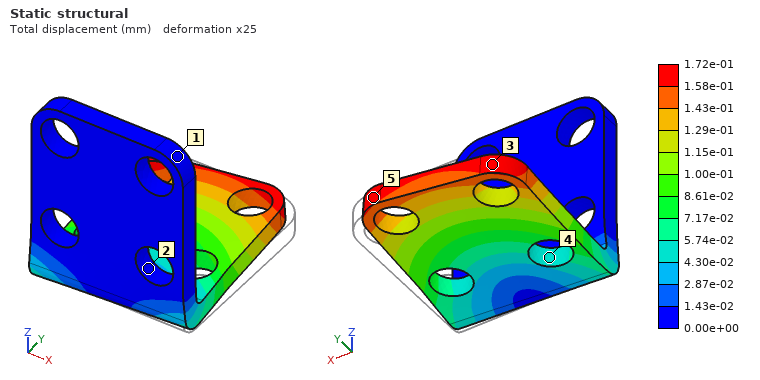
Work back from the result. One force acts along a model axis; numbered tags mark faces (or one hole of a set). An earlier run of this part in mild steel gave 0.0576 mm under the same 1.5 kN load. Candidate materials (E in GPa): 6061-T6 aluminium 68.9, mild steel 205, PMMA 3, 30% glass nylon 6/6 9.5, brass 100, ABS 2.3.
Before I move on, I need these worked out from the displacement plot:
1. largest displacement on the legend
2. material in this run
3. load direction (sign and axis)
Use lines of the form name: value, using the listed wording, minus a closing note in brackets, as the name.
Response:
largest displacement on the legend: 1.72e-01 mm
material in this run: 6061-T6 aluminium
load direction: -X
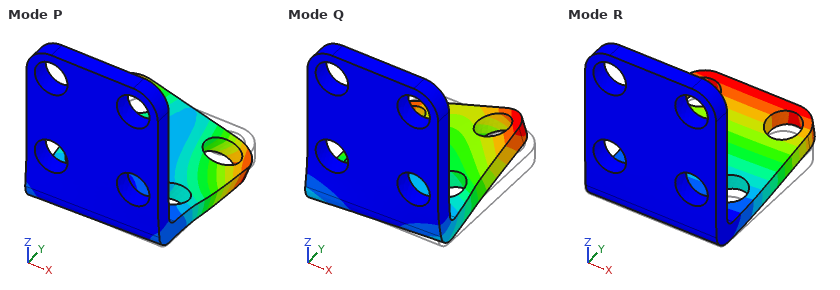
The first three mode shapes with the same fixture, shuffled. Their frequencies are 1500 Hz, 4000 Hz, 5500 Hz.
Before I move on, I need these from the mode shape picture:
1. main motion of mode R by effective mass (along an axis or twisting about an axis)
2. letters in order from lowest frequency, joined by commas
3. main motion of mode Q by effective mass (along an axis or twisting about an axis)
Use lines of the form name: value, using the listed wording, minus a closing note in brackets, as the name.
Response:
main motion of mode R by effective mass: along Z
letters in order from lowest frequency, joined by commas: R, Q, P
main motion of mode Q by effective mass: along X
